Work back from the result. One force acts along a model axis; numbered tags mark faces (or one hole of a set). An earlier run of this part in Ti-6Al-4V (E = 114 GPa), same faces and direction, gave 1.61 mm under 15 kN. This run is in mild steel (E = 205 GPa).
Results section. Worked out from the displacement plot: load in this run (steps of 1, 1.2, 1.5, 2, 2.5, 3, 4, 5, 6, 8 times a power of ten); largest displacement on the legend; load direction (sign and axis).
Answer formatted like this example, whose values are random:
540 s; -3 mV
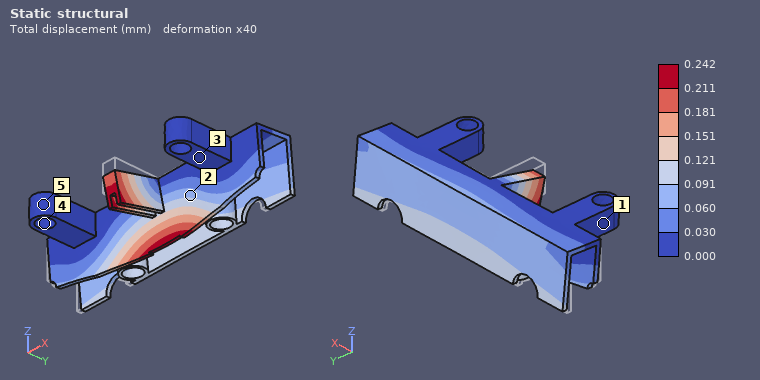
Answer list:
4 kN; 0.242 mm; +Y
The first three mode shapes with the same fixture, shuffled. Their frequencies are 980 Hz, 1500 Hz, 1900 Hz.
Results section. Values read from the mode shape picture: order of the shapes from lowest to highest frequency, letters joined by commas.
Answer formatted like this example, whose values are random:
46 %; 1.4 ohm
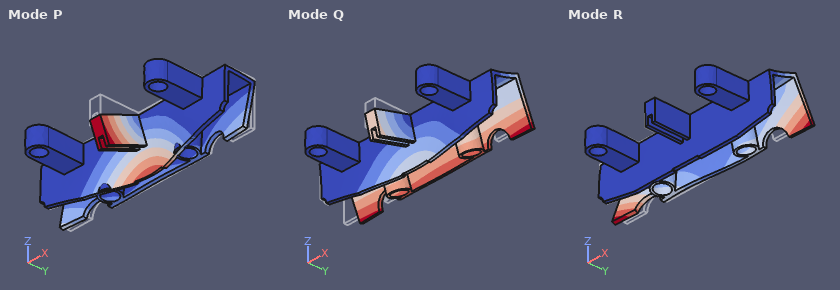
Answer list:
Q, R, P
